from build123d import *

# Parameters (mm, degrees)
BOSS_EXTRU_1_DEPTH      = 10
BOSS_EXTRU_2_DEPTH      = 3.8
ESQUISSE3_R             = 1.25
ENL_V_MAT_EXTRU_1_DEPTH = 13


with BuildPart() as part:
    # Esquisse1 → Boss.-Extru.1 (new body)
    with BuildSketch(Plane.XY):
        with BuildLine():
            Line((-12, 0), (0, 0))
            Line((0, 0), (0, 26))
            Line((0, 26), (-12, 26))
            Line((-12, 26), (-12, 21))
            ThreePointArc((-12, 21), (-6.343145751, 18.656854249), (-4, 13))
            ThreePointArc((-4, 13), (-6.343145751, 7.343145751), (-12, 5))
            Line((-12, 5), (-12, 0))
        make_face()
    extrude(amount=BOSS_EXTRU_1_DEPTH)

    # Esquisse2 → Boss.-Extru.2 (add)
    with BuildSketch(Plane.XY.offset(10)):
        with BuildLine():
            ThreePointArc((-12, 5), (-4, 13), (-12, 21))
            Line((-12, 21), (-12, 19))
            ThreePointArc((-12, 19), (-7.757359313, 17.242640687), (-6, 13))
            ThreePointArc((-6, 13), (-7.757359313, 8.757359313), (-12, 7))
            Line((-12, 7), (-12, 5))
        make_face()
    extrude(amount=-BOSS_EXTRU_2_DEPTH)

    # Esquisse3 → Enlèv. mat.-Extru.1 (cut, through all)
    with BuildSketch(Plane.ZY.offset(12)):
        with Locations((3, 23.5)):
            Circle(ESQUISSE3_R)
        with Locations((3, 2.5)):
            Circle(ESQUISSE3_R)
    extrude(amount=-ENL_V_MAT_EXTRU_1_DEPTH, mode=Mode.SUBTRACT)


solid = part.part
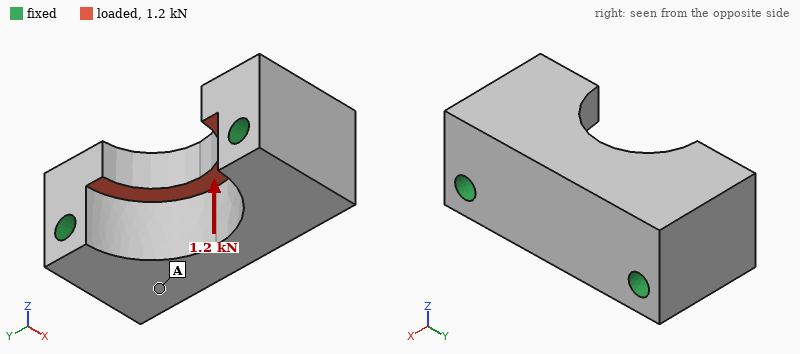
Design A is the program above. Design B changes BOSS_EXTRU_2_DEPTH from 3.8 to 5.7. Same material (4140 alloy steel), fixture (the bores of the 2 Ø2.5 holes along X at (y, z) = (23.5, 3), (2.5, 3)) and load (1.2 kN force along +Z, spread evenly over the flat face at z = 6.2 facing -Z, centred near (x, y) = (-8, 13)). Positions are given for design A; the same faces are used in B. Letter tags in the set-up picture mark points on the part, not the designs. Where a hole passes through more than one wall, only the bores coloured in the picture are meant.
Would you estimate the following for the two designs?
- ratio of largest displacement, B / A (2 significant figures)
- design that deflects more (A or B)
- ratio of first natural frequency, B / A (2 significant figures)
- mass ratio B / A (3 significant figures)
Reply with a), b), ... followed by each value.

a) 0.81
b) A
c) 0.99
d) 1.04
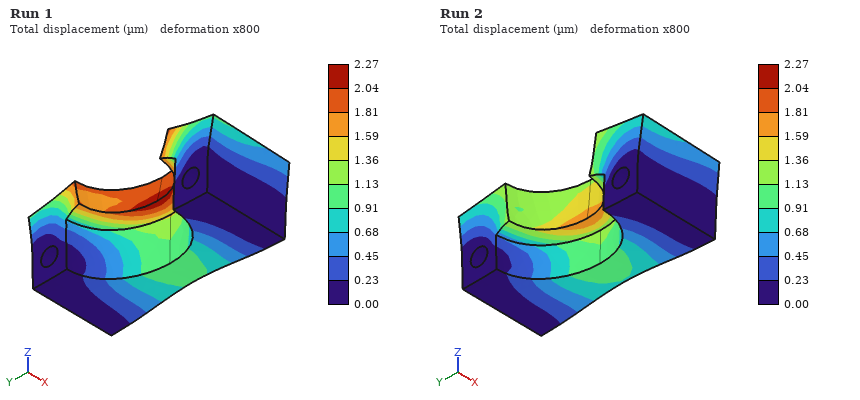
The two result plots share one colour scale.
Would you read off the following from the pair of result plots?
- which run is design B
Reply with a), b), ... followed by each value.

a) Run 2
